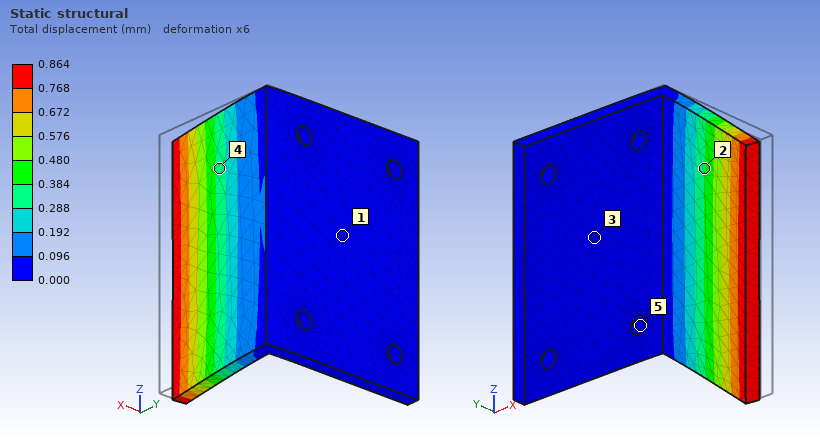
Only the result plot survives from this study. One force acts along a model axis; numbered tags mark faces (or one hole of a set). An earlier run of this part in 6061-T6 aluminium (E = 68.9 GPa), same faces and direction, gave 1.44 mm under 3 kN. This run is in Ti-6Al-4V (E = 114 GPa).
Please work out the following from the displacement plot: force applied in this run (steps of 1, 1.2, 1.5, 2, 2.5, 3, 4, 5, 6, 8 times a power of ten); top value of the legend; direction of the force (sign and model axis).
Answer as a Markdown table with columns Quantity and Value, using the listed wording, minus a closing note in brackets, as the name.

| Quantity | Value |
|---|---|
| force applied in this run | 3 kN |
| top value of the legend | 0.864 mm |
| direction of the force | -X |
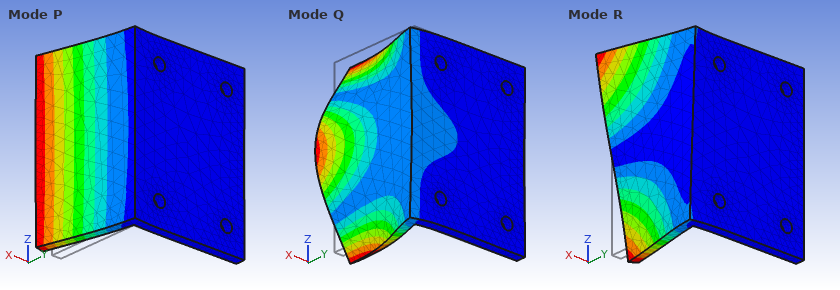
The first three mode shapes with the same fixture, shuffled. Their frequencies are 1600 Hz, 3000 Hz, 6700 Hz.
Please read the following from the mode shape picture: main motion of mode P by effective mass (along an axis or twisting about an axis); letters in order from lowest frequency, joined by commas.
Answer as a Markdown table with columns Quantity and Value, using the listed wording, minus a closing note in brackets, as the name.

| Quantity | Value |
|---|---|
| main motion of mode P by effective mass | along X |
| letters in order from lowest frequency, joined by commas | P, R, Q |
